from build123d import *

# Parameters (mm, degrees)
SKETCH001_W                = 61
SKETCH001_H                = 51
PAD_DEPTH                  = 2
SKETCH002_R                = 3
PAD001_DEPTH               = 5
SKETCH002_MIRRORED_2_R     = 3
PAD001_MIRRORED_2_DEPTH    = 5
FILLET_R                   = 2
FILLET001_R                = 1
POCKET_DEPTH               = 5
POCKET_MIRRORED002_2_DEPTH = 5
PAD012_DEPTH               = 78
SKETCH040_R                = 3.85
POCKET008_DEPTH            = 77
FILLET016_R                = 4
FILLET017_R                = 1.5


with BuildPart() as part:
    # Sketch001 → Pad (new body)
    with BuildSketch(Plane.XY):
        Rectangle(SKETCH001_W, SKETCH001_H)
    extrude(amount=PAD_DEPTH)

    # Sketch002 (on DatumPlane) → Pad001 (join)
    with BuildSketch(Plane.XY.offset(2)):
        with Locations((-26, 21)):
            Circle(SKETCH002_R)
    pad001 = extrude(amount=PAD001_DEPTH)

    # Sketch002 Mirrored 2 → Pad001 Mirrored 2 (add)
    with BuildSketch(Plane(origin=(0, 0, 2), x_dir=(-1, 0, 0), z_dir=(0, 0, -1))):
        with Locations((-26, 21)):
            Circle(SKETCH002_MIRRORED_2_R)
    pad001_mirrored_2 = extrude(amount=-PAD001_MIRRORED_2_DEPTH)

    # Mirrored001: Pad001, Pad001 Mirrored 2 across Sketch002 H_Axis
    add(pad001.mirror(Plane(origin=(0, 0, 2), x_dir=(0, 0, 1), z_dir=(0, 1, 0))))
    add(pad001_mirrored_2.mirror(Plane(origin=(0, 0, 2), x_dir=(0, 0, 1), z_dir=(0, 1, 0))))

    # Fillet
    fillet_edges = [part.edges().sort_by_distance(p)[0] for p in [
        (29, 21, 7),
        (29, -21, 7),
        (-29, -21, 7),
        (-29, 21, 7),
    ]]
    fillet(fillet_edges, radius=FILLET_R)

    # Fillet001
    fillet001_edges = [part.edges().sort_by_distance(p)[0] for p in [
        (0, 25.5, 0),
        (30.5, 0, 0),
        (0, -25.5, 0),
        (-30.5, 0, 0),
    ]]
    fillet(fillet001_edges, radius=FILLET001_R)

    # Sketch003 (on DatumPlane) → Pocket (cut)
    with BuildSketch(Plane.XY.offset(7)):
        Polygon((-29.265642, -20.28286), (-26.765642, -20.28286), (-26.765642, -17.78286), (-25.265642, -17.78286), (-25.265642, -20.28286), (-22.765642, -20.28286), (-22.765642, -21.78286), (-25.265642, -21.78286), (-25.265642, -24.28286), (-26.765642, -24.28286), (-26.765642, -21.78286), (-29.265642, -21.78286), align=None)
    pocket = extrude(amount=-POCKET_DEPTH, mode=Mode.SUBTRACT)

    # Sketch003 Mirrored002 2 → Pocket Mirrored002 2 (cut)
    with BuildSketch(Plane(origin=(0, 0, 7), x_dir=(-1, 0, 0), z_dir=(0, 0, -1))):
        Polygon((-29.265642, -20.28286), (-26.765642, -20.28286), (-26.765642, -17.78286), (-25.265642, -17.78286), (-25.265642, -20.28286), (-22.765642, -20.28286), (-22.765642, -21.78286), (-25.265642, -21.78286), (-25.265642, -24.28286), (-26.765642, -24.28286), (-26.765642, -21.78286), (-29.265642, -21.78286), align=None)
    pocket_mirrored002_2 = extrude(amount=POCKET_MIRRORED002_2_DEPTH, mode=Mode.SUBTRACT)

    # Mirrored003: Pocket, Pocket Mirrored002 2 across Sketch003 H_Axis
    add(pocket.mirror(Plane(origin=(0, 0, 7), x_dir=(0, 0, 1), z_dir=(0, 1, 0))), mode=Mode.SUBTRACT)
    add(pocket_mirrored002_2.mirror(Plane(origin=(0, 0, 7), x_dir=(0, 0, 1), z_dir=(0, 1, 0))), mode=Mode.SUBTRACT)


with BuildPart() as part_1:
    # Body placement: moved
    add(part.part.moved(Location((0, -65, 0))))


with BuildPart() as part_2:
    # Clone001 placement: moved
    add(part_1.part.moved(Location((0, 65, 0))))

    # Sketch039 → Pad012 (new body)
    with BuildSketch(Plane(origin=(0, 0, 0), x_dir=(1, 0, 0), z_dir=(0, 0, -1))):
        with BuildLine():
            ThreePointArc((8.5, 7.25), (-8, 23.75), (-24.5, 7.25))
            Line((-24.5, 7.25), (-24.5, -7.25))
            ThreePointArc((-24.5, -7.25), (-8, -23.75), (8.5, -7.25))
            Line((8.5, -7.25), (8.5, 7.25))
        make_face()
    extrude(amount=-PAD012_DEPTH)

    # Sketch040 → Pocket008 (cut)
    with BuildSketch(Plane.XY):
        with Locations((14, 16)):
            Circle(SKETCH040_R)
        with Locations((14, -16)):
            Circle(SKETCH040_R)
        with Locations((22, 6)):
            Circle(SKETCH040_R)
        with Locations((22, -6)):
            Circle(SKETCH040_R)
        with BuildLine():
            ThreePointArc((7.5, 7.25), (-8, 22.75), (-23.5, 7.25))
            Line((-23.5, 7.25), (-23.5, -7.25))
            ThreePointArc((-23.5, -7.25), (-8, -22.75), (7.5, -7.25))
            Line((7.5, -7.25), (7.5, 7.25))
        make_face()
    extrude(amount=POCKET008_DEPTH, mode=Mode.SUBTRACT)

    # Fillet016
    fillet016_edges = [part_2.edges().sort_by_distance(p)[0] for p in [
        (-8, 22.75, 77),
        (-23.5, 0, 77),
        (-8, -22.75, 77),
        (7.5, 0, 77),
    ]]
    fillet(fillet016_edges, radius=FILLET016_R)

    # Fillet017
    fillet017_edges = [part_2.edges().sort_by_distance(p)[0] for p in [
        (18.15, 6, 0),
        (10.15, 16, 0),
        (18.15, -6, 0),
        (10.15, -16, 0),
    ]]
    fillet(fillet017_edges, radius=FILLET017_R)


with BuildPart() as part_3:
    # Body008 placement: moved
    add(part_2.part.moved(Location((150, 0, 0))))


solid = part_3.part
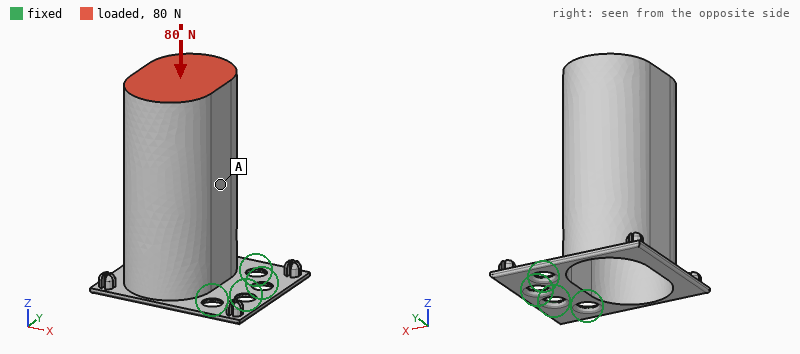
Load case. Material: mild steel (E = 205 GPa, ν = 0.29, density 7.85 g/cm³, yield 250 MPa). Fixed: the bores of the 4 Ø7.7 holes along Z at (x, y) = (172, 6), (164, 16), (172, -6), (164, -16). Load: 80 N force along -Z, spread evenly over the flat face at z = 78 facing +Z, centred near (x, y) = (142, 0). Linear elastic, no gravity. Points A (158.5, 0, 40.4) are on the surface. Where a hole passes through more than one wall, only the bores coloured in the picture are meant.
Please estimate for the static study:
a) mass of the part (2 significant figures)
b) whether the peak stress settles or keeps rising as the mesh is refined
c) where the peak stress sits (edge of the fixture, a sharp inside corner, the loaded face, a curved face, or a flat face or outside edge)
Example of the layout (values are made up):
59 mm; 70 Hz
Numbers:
120 g; keeps rising; edge of the fixture
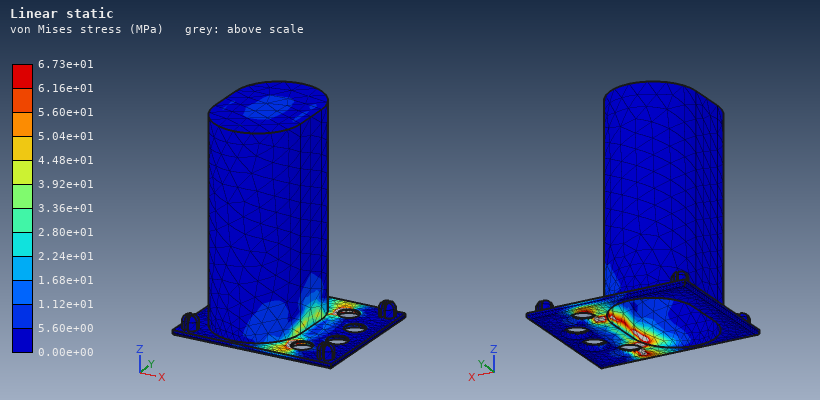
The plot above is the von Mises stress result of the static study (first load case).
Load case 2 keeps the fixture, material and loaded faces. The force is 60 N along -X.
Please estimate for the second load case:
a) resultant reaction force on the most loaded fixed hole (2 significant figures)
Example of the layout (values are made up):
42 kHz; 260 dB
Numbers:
220 N
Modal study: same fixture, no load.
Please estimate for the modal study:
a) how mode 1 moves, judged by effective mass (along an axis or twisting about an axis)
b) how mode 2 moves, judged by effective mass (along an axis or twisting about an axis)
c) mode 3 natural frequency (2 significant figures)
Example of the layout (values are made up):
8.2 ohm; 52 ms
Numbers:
along X; along Y; 2200 Hz
